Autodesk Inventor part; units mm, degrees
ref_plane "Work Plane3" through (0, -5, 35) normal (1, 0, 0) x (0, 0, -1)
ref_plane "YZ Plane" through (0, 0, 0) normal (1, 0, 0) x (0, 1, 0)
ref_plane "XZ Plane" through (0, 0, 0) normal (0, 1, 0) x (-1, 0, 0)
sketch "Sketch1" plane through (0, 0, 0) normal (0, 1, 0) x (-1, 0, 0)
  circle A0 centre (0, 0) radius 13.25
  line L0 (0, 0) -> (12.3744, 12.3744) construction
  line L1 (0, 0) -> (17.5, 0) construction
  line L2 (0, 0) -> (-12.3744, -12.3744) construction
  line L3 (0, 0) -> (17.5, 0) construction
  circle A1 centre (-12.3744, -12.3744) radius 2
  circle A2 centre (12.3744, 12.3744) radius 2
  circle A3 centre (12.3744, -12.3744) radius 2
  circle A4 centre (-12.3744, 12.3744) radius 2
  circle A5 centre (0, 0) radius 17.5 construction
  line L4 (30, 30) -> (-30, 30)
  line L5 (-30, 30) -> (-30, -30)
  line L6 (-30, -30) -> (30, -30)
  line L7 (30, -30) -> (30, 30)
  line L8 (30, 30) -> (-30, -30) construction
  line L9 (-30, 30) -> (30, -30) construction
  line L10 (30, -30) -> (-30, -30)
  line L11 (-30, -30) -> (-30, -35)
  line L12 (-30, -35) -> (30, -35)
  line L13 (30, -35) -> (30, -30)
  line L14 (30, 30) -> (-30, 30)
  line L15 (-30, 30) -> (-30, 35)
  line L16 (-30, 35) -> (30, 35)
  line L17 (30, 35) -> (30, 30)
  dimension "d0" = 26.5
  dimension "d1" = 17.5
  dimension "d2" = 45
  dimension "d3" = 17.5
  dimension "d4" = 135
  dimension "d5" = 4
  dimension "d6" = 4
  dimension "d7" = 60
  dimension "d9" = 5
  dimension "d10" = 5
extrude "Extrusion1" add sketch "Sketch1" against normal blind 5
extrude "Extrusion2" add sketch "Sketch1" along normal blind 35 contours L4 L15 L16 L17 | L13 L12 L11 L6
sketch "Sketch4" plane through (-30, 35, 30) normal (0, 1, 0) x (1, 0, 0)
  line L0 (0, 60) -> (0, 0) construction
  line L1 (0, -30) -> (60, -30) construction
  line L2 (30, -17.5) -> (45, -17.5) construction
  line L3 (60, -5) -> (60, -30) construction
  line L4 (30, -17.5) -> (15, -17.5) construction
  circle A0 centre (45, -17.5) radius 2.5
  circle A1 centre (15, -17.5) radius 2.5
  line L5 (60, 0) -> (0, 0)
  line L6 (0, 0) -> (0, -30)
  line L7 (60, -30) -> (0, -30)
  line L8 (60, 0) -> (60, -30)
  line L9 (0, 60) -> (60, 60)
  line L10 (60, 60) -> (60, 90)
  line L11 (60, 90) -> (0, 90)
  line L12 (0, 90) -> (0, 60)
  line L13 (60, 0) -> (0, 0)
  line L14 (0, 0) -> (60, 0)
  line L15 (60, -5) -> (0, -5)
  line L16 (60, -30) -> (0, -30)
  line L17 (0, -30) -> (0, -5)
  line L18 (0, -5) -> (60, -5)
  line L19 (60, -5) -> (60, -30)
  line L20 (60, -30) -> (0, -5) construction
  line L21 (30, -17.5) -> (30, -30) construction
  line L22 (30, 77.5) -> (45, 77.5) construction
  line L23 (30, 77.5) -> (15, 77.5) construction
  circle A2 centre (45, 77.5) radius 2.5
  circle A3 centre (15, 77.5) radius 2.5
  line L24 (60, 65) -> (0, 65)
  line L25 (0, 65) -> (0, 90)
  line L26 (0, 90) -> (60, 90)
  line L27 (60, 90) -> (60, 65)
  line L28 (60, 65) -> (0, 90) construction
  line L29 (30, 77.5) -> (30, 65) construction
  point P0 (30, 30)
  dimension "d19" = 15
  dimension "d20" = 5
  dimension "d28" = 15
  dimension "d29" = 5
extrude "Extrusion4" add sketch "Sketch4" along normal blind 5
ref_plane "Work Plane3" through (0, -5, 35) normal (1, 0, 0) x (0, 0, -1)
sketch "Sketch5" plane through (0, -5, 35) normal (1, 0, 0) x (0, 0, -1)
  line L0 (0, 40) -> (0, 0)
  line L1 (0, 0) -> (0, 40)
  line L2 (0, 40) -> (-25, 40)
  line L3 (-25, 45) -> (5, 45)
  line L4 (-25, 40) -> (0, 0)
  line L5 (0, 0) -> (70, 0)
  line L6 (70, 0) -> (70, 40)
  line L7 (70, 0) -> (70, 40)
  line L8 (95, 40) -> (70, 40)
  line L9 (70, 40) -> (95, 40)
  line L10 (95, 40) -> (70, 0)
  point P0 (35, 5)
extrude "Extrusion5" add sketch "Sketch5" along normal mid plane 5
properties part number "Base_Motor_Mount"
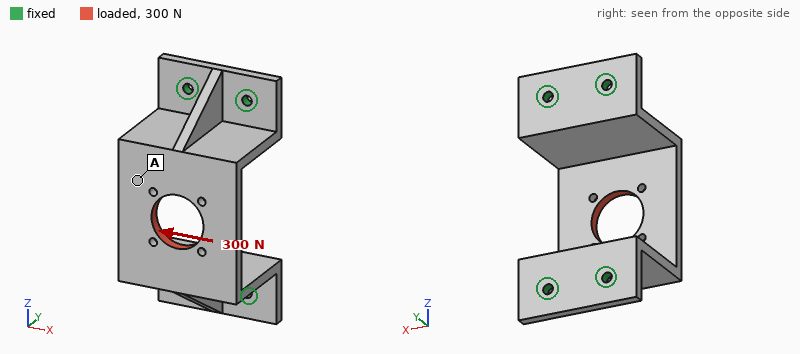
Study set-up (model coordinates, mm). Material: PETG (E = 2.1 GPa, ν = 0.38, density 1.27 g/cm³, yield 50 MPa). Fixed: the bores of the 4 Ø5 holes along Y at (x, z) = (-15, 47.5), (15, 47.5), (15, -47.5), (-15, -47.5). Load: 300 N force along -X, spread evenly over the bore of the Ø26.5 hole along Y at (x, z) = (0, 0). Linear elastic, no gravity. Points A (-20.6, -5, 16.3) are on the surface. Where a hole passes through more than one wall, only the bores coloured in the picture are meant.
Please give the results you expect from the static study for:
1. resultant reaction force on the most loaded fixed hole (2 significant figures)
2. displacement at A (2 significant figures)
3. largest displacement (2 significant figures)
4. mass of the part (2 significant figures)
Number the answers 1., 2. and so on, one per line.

1. 210 N
2. 0.46 mm
3. 0.50 mm
4. 78 g
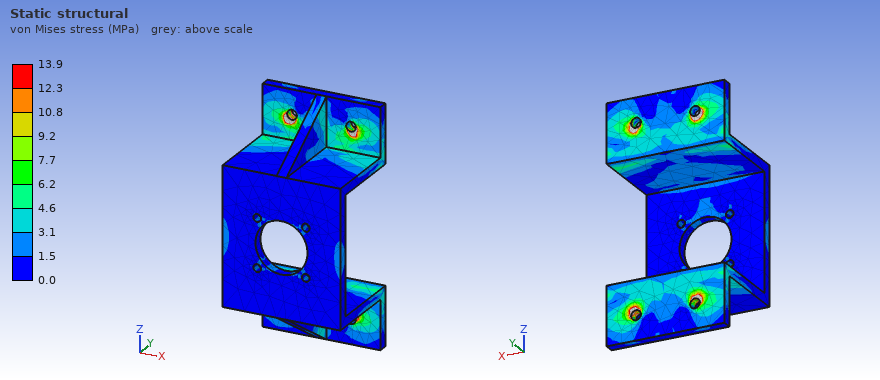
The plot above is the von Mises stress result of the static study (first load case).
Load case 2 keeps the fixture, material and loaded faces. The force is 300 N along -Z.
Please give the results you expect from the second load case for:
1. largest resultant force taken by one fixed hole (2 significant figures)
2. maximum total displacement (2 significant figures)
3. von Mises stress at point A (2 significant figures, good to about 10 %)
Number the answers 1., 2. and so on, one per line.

1. 81 N
2. 0.70 mm
3. 4.2 MPa
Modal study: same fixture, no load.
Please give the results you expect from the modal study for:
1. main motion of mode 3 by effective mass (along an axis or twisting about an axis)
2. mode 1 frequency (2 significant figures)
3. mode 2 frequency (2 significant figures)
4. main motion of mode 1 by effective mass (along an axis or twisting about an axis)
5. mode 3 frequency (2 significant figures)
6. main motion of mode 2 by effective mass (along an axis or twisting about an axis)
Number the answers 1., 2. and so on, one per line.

1. twisting about Y
2. 550 Hz
3. 680 Hz
4. along Z
5. 770 Hz
6. along X
